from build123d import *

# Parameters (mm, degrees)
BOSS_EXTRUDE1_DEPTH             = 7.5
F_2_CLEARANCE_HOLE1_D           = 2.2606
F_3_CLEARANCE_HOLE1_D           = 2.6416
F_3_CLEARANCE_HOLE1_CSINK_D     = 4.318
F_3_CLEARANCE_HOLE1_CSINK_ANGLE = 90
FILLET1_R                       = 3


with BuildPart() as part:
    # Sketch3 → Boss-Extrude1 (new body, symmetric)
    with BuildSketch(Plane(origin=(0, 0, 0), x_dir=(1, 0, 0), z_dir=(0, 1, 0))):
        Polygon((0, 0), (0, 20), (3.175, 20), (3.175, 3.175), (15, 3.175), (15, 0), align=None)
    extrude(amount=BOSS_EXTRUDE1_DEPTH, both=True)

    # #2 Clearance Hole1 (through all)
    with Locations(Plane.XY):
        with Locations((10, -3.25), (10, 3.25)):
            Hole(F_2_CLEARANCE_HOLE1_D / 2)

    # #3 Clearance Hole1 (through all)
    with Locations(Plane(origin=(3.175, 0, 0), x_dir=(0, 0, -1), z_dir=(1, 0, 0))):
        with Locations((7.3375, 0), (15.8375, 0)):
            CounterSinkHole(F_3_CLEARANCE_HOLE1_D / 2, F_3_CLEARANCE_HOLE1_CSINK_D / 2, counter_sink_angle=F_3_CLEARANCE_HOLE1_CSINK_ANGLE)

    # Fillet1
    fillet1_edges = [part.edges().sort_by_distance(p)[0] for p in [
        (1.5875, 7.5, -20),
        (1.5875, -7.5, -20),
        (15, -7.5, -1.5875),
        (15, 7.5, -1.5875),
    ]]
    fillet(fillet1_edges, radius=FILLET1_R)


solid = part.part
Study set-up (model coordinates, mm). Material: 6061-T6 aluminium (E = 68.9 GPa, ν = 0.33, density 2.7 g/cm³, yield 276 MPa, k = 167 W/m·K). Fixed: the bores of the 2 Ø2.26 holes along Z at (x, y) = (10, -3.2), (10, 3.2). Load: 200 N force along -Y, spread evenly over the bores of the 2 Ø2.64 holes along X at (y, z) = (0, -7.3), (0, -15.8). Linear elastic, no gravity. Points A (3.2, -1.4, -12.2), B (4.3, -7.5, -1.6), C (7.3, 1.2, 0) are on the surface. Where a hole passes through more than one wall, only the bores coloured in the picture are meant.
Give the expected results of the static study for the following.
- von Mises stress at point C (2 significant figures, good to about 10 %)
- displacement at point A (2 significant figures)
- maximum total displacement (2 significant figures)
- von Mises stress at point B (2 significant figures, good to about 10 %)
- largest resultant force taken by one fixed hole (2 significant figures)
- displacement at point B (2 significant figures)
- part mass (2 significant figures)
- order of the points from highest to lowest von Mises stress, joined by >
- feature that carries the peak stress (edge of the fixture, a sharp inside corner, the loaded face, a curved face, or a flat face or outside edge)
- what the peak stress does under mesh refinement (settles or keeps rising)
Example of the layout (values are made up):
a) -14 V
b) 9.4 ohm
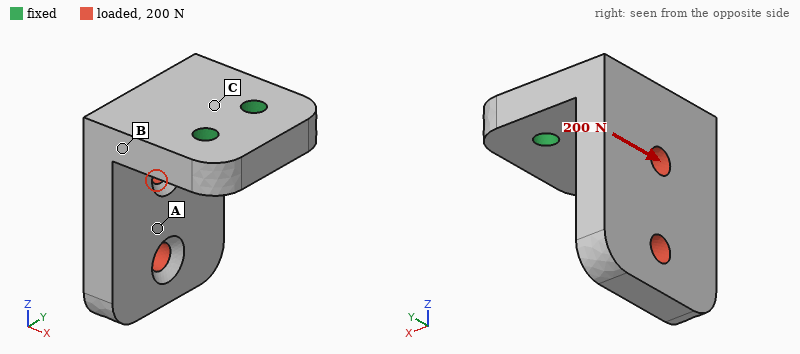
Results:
a) 25 MPa
b) 29 µm
c) 49 µm
d) 47 MPa
e) 300 N
f) 12 µm
g) 3.8 g
h) B > C > A
i) edge of the fixture
j) keeps rising
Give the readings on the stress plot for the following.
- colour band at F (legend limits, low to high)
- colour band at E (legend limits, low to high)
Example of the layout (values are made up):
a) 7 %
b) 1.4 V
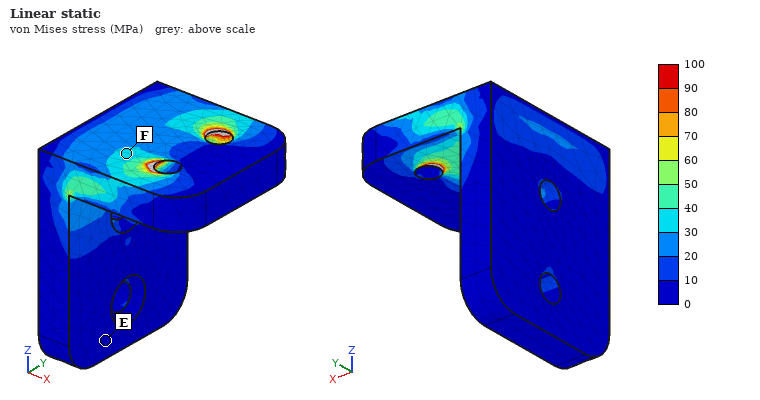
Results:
a) 30 to 40 MPa
b) 0 to 10 MPa
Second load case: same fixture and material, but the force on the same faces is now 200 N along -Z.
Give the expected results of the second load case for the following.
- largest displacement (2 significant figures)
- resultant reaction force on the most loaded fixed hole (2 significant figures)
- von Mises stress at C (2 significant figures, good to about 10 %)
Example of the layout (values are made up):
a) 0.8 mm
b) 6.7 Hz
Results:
a) 56 µm
b) 100 N
c) 42 MPa
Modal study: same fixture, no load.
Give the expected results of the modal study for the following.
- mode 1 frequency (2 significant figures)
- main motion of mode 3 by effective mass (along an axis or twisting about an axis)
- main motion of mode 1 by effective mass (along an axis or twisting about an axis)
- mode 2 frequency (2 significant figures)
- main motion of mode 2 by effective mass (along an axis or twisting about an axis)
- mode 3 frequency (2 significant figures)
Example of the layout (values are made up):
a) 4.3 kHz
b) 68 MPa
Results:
a) 4800 Hz
b) along Z
c) along X
d) 8200 Hz
e) along Y
f) 16 kHz
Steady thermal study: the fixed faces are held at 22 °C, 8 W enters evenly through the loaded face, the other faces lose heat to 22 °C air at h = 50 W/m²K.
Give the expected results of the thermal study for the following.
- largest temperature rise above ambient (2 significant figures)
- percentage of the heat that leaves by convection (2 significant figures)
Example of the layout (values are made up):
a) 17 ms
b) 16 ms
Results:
a) 18 K
b) 6.5 %
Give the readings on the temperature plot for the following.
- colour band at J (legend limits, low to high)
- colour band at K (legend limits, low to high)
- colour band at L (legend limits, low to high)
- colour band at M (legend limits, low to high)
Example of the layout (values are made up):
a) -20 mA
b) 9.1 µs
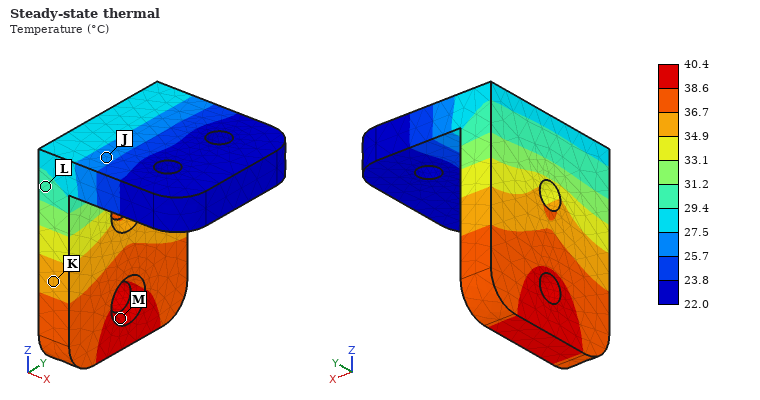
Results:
a) 25.7 to 27.5 °C
b) 34.9 to 36.7 °C
c) 29.4 to 31.2 °C
d) 38.6 to 40.4 °C
